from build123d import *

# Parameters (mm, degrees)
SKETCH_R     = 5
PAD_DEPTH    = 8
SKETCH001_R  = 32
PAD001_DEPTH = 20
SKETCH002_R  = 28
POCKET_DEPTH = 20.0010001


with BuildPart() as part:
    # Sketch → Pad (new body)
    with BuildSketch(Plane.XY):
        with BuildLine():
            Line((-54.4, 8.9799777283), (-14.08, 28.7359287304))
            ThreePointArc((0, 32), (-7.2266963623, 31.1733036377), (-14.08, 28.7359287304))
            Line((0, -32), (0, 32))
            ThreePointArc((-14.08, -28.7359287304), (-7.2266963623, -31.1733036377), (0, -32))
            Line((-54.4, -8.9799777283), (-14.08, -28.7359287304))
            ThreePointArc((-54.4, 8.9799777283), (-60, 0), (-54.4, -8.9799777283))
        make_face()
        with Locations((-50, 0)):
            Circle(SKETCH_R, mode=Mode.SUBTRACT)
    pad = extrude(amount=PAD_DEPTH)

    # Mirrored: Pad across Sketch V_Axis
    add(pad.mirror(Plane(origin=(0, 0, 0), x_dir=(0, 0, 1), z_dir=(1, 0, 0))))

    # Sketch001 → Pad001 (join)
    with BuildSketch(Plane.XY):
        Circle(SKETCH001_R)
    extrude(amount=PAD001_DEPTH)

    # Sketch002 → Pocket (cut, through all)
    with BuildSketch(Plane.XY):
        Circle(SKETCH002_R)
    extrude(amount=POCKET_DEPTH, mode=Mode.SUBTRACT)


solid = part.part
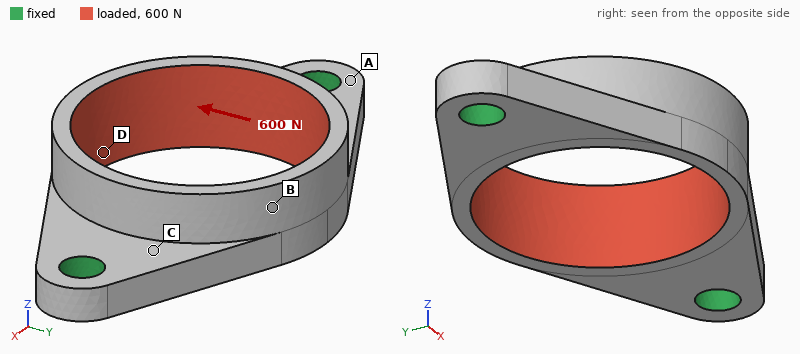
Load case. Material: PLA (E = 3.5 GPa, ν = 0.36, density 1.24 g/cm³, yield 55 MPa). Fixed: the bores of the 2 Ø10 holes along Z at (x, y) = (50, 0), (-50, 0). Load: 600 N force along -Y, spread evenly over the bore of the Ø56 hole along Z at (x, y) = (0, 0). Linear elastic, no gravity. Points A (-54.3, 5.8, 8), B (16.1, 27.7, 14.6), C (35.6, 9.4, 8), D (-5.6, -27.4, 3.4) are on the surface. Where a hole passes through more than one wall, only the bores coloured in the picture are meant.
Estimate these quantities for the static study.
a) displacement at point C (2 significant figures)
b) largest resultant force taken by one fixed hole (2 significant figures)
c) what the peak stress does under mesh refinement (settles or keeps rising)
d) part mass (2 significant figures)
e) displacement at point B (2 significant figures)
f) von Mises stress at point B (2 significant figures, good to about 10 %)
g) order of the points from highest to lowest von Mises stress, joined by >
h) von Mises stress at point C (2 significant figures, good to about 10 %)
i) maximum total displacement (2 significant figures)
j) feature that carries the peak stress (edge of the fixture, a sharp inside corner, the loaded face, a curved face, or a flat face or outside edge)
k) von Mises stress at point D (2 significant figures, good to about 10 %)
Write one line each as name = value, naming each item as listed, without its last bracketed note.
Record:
displacement at point C = 0.053 mm
largest resultant force taken by one fixed hole = 300 N
what the peak stress does under mesh refinement = keeps rising
part mass = 34 g
displacement at point B = 0.22 mm
von Mises stress at point B = 2.3 MPa
order of the points from highest to lowest von Mises stress, joined by > = C > D > B > A
von Mises stress at point C = 5.4 MPa
maximum total displacement = 0.29 mm
feature that carries the peak stress = edge of the fixture
von Mises stress at point D = 3.6 MPa
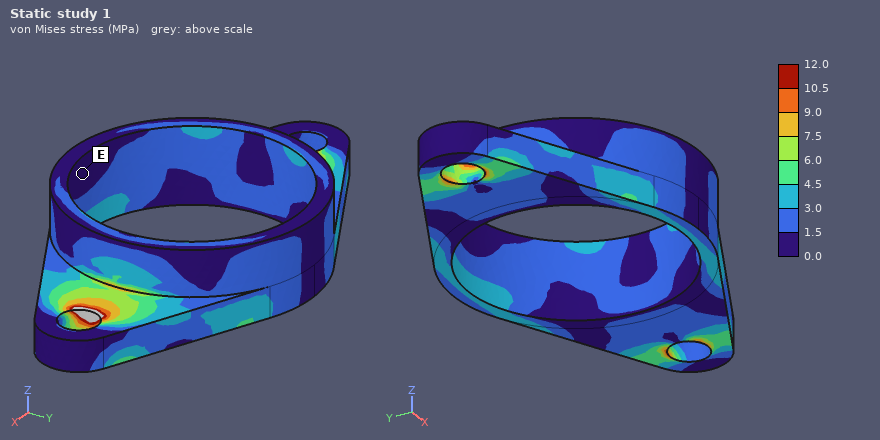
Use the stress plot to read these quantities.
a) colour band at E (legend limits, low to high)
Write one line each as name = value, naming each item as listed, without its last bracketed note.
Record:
colour band at E = 0.0 to 1.5 MPa
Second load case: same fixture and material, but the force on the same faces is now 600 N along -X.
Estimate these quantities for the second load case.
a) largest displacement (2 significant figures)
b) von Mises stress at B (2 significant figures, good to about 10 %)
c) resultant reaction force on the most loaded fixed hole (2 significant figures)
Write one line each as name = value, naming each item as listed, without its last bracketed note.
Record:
largest displacement = 62 µm
von Mises stress at B = 2.0 MPa
resultant reaction force on the most loaded fixed hole = 300 N
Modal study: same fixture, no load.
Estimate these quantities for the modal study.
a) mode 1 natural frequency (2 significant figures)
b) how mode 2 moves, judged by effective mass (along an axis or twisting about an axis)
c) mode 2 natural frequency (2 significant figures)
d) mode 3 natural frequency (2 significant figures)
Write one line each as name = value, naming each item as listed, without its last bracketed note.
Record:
mode 1 natural frequency = 1100 Hz
how mode 2 moves, judged by effective mass = along Z
mode 2 natural frequency = 1400 Hz
mode 3 natural frequency = 2300 Hz
